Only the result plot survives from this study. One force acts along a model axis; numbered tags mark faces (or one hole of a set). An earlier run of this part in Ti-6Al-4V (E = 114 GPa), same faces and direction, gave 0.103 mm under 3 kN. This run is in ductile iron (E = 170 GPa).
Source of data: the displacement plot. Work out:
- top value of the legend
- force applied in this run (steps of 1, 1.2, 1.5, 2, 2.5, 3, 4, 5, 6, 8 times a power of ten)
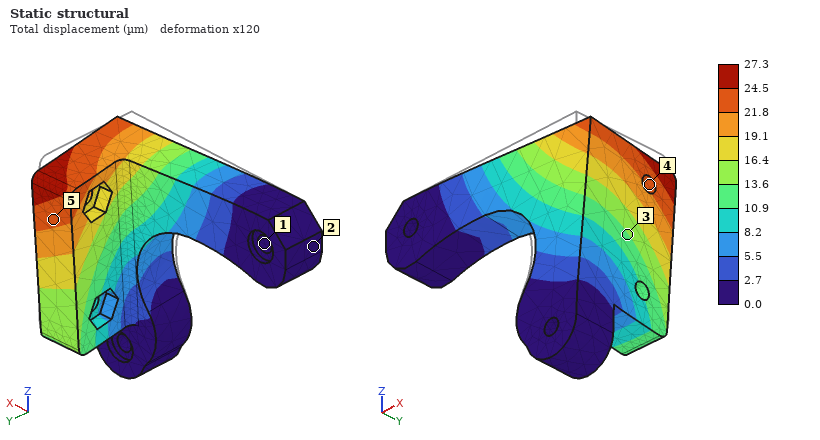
27.3 µm
1.2 kN
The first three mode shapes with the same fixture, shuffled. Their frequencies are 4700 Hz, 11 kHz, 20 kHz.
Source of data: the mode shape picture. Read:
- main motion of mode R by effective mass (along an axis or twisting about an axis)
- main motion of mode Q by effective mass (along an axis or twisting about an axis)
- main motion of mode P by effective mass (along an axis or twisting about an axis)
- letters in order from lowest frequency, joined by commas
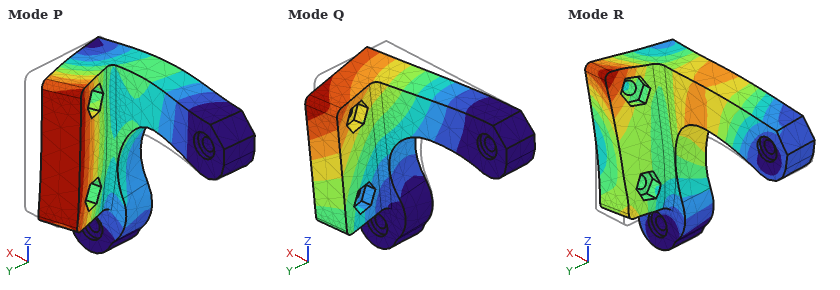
along Z
along Y
along X
Q, P, R
